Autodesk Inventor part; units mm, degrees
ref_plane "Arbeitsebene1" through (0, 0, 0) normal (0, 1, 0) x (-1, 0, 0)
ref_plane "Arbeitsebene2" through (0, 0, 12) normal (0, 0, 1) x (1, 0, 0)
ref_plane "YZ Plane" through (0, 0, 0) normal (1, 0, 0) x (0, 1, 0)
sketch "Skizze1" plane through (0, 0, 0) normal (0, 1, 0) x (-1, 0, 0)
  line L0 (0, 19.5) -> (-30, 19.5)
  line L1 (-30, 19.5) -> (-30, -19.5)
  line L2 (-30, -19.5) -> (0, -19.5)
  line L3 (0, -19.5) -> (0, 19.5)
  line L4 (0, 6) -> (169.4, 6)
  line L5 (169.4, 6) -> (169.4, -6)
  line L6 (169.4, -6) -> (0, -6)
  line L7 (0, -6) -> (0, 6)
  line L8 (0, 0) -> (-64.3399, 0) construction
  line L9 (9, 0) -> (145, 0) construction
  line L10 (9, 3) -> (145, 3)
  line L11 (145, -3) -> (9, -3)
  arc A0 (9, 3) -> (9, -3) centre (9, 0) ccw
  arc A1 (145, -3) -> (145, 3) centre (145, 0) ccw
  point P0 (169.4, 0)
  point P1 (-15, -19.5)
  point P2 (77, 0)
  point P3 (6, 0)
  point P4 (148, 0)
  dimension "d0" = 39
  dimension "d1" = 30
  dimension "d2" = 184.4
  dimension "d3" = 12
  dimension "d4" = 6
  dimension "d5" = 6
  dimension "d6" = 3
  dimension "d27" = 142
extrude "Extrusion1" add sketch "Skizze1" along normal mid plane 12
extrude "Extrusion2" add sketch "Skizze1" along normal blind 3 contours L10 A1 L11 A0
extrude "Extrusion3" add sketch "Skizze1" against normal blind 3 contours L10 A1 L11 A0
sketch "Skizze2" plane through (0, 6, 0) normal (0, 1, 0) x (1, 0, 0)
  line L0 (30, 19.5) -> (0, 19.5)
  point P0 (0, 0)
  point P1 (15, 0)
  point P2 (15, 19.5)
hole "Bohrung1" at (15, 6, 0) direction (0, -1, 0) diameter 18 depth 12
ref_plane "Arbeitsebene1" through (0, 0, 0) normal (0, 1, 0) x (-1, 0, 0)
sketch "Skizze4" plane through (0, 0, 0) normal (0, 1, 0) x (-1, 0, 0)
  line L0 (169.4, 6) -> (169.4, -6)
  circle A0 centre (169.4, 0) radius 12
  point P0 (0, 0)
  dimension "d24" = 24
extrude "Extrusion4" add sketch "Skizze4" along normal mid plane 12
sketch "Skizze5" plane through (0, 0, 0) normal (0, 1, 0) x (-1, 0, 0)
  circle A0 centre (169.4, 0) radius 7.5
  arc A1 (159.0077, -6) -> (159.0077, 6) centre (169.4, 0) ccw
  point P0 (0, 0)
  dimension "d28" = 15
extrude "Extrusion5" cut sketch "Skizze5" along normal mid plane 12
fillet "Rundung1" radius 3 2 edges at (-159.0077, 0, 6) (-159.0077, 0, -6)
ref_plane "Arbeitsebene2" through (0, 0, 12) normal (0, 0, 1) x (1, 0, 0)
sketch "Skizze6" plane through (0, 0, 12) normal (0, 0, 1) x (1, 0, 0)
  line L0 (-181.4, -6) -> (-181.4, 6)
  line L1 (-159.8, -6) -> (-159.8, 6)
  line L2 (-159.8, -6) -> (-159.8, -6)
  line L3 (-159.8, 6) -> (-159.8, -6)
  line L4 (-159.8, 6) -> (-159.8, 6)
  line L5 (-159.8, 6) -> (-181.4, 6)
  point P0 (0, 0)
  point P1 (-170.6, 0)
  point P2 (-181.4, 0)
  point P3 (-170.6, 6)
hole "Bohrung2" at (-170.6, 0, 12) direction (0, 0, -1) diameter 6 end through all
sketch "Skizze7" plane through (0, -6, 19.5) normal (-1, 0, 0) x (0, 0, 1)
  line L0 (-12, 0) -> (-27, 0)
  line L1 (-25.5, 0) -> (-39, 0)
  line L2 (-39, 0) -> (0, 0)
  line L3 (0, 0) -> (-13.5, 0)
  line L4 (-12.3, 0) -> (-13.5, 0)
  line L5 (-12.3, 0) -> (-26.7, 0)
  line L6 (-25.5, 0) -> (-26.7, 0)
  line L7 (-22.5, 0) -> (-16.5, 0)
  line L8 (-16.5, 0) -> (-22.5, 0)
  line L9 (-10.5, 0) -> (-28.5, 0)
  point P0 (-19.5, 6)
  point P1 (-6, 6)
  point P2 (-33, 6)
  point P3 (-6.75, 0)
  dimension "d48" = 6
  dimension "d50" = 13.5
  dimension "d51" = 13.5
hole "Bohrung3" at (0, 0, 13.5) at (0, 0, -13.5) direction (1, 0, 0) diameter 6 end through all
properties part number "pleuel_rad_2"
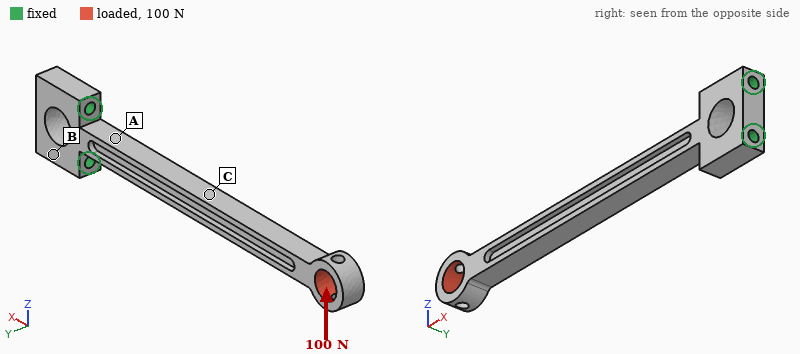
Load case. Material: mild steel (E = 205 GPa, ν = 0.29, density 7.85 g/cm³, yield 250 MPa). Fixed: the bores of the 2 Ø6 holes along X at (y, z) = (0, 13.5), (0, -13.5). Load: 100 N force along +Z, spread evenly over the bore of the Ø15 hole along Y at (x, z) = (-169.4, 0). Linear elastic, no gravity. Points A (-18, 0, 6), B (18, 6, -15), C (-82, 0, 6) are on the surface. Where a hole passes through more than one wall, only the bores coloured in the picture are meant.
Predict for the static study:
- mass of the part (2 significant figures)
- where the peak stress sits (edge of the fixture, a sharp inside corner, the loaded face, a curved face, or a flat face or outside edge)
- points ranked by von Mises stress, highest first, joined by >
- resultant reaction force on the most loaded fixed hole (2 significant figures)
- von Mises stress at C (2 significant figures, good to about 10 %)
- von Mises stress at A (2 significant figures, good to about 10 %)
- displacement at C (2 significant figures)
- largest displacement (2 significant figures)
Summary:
240 g
a flat face or outside edge
A > C > B
1.1 kN
32 MPa
56 MPa
0.17 mm
0.58 mm
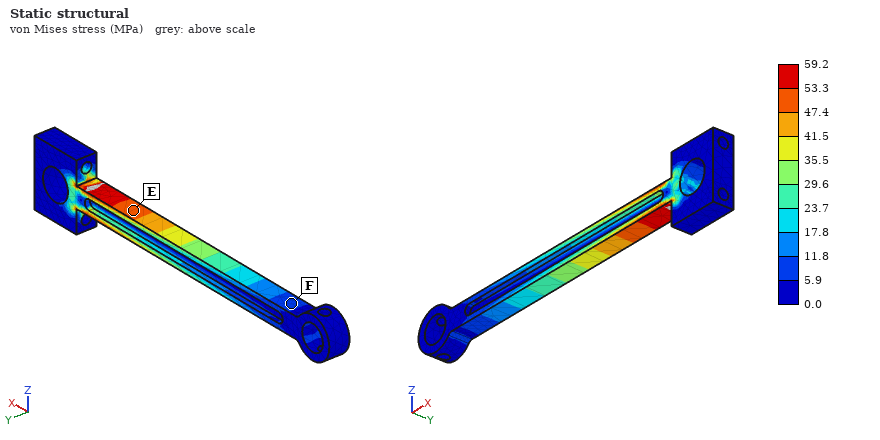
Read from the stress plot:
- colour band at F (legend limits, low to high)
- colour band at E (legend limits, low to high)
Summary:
5.9 to 11.8 MPa
47.4 to 53.3 MPa
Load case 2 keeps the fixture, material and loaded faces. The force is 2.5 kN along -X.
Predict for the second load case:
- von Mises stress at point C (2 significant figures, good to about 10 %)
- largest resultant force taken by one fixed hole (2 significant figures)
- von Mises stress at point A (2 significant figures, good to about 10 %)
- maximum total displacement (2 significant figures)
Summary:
23 MPa
1.4 kN
23 MPa
27 µm
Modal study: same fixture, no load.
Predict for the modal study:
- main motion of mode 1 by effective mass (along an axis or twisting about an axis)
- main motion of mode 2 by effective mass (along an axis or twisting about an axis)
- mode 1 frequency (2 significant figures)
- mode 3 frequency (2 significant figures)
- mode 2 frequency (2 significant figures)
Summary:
along Y
along Z
230 Hz
1500 Hz
300 Hz
